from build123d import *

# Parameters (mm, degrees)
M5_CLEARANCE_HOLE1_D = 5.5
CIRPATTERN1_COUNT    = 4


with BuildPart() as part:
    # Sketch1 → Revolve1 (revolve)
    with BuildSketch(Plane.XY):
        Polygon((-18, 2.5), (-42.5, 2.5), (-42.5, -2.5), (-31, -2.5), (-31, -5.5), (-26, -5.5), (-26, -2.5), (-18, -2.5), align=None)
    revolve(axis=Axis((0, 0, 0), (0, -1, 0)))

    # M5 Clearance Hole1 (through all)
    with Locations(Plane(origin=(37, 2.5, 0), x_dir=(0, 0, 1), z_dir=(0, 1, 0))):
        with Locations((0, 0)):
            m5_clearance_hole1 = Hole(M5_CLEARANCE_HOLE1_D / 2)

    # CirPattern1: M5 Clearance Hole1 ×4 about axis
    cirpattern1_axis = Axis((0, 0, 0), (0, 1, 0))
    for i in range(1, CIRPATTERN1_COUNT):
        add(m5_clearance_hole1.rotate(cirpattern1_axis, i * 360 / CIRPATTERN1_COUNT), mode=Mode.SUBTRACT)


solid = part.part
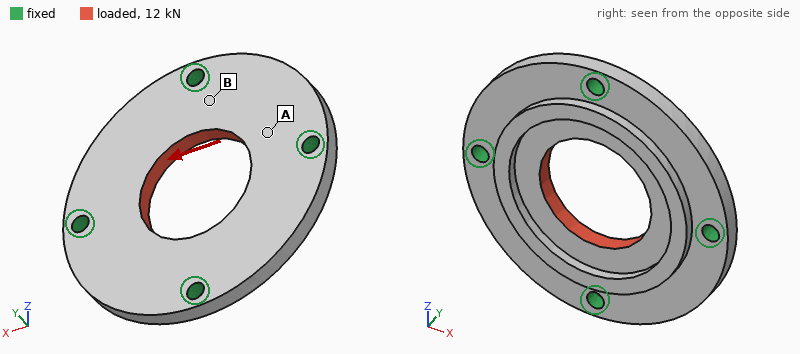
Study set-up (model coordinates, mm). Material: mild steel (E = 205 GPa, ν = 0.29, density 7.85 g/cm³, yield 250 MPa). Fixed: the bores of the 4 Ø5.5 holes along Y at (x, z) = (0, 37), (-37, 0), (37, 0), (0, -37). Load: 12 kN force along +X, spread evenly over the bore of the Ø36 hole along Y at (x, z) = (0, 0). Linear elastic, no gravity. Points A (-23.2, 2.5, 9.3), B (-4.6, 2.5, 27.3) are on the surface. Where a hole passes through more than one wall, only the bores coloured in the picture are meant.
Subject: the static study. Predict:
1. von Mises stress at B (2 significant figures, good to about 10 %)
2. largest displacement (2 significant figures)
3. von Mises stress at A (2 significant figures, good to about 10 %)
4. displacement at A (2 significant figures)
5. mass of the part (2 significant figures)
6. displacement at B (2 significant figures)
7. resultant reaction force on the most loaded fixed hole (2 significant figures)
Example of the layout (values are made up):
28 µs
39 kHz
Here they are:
13 MPa
5.1 µm
31 MPa
3.2 µm
200 g
2.5 µm
3.3 kN
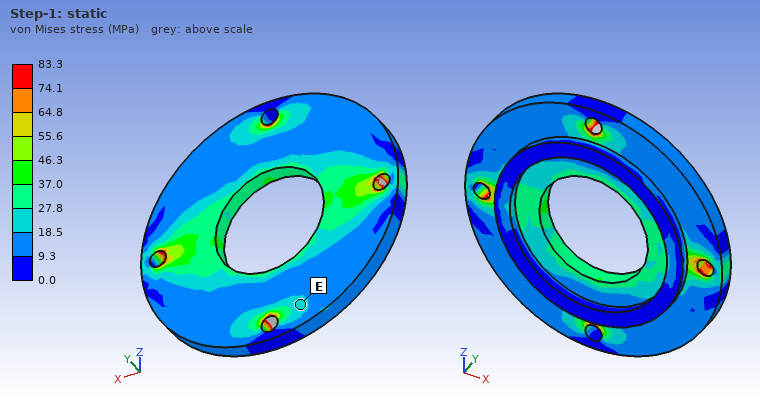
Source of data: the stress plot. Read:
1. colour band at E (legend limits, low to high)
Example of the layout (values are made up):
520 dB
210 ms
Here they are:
18.5 to 27.8 MPa
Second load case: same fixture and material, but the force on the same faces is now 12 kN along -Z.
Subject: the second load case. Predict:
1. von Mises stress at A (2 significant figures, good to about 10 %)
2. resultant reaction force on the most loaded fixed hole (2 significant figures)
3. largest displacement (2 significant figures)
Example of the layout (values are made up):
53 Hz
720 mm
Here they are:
13 MPa
3.3 kN
5.1 µm
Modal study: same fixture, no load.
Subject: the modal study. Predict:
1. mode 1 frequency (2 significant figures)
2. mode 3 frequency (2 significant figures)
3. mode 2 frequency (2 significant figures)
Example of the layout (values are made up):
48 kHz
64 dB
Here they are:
8200 Hz
9100 Hz
9100 Hz
